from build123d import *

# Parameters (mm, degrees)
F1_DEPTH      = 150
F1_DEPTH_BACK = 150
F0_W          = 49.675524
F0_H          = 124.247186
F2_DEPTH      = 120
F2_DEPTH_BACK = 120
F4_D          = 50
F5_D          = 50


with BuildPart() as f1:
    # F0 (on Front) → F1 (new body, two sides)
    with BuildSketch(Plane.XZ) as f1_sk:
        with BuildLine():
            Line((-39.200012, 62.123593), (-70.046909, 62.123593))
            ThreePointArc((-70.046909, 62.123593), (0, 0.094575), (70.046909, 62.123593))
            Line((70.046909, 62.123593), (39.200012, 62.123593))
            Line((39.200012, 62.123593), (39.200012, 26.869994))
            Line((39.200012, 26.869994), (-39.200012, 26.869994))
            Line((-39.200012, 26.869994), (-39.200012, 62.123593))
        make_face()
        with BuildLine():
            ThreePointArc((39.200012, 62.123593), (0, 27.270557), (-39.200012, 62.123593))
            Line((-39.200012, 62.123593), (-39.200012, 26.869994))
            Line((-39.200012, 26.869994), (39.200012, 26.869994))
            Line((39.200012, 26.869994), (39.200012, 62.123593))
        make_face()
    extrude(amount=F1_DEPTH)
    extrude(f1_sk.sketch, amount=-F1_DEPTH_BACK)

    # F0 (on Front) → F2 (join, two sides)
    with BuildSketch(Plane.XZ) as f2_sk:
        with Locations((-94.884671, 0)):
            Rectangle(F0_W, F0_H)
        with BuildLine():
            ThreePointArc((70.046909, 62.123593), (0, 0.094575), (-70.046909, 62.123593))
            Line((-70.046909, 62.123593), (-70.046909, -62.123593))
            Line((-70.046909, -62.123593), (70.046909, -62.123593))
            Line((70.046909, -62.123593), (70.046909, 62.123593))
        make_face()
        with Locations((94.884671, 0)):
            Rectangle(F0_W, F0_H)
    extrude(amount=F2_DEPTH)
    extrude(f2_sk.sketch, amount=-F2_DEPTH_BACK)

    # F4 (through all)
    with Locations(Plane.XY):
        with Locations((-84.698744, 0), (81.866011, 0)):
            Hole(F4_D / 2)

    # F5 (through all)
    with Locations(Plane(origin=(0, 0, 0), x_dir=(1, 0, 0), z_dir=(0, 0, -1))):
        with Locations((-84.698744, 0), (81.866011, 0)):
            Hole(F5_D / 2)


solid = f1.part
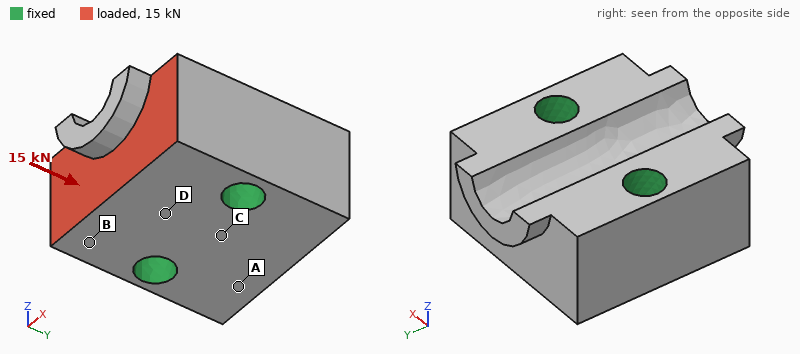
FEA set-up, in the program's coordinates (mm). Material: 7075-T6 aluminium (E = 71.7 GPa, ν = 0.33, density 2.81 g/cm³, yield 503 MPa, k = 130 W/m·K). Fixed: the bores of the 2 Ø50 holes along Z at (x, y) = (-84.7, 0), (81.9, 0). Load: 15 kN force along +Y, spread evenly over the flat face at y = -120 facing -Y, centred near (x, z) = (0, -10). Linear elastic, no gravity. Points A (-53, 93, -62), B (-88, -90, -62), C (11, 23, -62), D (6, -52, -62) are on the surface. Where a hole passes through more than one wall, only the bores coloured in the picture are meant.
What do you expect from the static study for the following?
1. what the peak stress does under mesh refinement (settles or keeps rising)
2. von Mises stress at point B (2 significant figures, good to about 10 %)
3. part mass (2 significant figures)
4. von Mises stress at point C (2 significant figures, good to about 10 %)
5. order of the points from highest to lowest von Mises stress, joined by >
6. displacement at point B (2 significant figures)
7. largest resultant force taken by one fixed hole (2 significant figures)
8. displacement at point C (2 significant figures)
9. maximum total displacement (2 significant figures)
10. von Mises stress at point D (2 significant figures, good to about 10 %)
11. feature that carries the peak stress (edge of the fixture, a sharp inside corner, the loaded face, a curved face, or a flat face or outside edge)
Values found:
keeps rising
0.70 MPa
18 kg
0.23 MPa
B > D > C > A
0.90 µm
7.6 kN
0.31 µm
1.3 µm
0.45 MPa
edge of the fixture
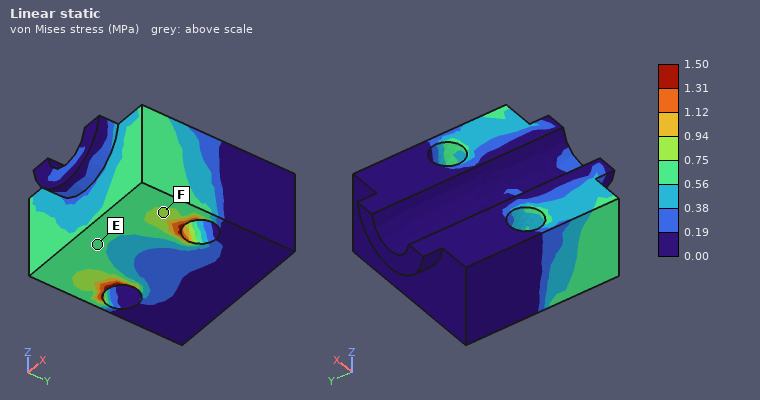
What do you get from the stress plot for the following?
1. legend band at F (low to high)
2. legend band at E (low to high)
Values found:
0.75 to 0.94 MPa
0.56 to 0.75 MPa
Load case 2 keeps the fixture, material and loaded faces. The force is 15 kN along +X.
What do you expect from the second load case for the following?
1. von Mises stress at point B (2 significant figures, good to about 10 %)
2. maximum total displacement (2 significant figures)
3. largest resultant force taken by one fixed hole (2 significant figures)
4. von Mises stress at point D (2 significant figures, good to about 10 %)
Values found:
0.81 MPa
4.8 µm
11 kN
1.4 MPa
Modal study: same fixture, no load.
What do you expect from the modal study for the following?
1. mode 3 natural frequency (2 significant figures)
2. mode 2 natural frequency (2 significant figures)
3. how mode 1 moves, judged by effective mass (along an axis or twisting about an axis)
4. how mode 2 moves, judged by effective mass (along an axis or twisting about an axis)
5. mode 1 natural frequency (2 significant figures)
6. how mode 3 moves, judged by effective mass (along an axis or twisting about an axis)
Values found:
5400 Hz
4700 Hz
twisting about X
along Z
4400 Hz
twisting about Z
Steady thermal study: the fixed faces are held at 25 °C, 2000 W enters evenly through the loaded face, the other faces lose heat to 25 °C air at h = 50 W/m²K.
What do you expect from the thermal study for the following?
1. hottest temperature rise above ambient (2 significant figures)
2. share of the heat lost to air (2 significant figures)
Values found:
62 K
8.1 %
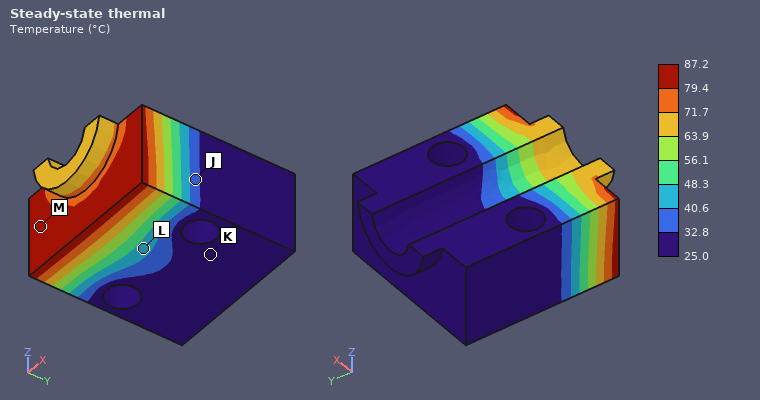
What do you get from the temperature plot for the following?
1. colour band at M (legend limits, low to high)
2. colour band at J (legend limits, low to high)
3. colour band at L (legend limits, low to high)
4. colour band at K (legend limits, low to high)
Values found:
79.4 to 87.2 °C
32.8 to 40.6 °C
40.6 to 48.3 °C
25.0 to 32.8 °C
